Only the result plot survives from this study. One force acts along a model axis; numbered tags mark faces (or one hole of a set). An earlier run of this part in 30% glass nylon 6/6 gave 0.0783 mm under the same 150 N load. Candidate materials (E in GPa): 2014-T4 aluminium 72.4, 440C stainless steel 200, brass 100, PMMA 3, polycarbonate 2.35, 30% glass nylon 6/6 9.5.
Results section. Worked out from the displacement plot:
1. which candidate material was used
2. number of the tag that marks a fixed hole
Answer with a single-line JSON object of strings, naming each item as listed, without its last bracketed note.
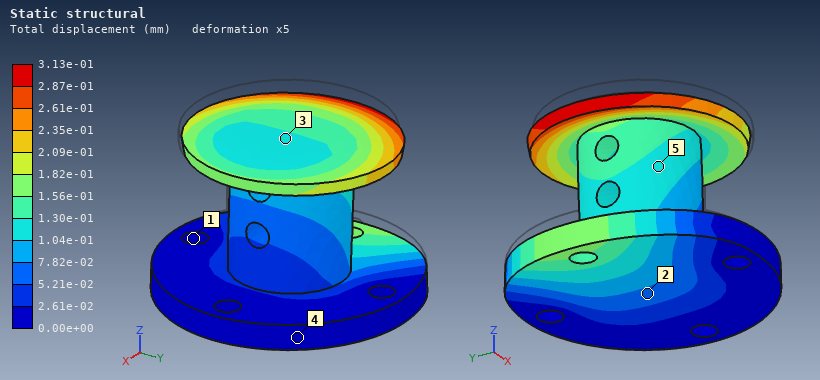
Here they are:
{"which candidate material was used": "polycarbonate", "number of the tag that marks a fixed hole": "1"}
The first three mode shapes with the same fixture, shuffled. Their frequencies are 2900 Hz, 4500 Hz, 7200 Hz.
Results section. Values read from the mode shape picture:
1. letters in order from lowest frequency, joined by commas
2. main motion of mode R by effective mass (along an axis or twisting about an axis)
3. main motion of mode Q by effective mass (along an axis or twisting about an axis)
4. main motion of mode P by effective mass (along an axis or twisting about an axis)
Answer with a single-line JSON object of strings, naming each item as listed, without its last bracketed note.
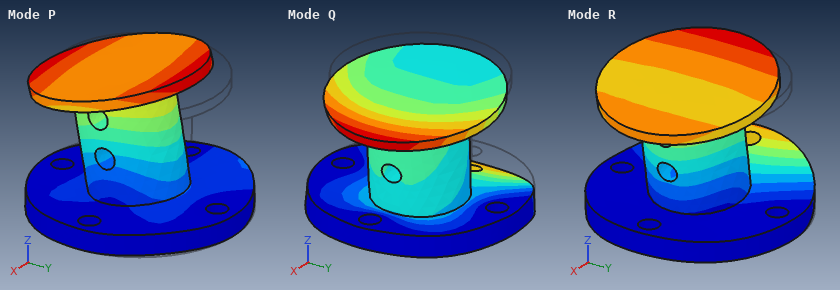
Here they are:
{"letters in order from lowest frequency, joined by commas": "R, P, Q", "main motion of mode R by effective mass": "along X", "main motion of mode Q by effective mass": "along Z", "main motion of mode P by effective mass": "along Y"}
